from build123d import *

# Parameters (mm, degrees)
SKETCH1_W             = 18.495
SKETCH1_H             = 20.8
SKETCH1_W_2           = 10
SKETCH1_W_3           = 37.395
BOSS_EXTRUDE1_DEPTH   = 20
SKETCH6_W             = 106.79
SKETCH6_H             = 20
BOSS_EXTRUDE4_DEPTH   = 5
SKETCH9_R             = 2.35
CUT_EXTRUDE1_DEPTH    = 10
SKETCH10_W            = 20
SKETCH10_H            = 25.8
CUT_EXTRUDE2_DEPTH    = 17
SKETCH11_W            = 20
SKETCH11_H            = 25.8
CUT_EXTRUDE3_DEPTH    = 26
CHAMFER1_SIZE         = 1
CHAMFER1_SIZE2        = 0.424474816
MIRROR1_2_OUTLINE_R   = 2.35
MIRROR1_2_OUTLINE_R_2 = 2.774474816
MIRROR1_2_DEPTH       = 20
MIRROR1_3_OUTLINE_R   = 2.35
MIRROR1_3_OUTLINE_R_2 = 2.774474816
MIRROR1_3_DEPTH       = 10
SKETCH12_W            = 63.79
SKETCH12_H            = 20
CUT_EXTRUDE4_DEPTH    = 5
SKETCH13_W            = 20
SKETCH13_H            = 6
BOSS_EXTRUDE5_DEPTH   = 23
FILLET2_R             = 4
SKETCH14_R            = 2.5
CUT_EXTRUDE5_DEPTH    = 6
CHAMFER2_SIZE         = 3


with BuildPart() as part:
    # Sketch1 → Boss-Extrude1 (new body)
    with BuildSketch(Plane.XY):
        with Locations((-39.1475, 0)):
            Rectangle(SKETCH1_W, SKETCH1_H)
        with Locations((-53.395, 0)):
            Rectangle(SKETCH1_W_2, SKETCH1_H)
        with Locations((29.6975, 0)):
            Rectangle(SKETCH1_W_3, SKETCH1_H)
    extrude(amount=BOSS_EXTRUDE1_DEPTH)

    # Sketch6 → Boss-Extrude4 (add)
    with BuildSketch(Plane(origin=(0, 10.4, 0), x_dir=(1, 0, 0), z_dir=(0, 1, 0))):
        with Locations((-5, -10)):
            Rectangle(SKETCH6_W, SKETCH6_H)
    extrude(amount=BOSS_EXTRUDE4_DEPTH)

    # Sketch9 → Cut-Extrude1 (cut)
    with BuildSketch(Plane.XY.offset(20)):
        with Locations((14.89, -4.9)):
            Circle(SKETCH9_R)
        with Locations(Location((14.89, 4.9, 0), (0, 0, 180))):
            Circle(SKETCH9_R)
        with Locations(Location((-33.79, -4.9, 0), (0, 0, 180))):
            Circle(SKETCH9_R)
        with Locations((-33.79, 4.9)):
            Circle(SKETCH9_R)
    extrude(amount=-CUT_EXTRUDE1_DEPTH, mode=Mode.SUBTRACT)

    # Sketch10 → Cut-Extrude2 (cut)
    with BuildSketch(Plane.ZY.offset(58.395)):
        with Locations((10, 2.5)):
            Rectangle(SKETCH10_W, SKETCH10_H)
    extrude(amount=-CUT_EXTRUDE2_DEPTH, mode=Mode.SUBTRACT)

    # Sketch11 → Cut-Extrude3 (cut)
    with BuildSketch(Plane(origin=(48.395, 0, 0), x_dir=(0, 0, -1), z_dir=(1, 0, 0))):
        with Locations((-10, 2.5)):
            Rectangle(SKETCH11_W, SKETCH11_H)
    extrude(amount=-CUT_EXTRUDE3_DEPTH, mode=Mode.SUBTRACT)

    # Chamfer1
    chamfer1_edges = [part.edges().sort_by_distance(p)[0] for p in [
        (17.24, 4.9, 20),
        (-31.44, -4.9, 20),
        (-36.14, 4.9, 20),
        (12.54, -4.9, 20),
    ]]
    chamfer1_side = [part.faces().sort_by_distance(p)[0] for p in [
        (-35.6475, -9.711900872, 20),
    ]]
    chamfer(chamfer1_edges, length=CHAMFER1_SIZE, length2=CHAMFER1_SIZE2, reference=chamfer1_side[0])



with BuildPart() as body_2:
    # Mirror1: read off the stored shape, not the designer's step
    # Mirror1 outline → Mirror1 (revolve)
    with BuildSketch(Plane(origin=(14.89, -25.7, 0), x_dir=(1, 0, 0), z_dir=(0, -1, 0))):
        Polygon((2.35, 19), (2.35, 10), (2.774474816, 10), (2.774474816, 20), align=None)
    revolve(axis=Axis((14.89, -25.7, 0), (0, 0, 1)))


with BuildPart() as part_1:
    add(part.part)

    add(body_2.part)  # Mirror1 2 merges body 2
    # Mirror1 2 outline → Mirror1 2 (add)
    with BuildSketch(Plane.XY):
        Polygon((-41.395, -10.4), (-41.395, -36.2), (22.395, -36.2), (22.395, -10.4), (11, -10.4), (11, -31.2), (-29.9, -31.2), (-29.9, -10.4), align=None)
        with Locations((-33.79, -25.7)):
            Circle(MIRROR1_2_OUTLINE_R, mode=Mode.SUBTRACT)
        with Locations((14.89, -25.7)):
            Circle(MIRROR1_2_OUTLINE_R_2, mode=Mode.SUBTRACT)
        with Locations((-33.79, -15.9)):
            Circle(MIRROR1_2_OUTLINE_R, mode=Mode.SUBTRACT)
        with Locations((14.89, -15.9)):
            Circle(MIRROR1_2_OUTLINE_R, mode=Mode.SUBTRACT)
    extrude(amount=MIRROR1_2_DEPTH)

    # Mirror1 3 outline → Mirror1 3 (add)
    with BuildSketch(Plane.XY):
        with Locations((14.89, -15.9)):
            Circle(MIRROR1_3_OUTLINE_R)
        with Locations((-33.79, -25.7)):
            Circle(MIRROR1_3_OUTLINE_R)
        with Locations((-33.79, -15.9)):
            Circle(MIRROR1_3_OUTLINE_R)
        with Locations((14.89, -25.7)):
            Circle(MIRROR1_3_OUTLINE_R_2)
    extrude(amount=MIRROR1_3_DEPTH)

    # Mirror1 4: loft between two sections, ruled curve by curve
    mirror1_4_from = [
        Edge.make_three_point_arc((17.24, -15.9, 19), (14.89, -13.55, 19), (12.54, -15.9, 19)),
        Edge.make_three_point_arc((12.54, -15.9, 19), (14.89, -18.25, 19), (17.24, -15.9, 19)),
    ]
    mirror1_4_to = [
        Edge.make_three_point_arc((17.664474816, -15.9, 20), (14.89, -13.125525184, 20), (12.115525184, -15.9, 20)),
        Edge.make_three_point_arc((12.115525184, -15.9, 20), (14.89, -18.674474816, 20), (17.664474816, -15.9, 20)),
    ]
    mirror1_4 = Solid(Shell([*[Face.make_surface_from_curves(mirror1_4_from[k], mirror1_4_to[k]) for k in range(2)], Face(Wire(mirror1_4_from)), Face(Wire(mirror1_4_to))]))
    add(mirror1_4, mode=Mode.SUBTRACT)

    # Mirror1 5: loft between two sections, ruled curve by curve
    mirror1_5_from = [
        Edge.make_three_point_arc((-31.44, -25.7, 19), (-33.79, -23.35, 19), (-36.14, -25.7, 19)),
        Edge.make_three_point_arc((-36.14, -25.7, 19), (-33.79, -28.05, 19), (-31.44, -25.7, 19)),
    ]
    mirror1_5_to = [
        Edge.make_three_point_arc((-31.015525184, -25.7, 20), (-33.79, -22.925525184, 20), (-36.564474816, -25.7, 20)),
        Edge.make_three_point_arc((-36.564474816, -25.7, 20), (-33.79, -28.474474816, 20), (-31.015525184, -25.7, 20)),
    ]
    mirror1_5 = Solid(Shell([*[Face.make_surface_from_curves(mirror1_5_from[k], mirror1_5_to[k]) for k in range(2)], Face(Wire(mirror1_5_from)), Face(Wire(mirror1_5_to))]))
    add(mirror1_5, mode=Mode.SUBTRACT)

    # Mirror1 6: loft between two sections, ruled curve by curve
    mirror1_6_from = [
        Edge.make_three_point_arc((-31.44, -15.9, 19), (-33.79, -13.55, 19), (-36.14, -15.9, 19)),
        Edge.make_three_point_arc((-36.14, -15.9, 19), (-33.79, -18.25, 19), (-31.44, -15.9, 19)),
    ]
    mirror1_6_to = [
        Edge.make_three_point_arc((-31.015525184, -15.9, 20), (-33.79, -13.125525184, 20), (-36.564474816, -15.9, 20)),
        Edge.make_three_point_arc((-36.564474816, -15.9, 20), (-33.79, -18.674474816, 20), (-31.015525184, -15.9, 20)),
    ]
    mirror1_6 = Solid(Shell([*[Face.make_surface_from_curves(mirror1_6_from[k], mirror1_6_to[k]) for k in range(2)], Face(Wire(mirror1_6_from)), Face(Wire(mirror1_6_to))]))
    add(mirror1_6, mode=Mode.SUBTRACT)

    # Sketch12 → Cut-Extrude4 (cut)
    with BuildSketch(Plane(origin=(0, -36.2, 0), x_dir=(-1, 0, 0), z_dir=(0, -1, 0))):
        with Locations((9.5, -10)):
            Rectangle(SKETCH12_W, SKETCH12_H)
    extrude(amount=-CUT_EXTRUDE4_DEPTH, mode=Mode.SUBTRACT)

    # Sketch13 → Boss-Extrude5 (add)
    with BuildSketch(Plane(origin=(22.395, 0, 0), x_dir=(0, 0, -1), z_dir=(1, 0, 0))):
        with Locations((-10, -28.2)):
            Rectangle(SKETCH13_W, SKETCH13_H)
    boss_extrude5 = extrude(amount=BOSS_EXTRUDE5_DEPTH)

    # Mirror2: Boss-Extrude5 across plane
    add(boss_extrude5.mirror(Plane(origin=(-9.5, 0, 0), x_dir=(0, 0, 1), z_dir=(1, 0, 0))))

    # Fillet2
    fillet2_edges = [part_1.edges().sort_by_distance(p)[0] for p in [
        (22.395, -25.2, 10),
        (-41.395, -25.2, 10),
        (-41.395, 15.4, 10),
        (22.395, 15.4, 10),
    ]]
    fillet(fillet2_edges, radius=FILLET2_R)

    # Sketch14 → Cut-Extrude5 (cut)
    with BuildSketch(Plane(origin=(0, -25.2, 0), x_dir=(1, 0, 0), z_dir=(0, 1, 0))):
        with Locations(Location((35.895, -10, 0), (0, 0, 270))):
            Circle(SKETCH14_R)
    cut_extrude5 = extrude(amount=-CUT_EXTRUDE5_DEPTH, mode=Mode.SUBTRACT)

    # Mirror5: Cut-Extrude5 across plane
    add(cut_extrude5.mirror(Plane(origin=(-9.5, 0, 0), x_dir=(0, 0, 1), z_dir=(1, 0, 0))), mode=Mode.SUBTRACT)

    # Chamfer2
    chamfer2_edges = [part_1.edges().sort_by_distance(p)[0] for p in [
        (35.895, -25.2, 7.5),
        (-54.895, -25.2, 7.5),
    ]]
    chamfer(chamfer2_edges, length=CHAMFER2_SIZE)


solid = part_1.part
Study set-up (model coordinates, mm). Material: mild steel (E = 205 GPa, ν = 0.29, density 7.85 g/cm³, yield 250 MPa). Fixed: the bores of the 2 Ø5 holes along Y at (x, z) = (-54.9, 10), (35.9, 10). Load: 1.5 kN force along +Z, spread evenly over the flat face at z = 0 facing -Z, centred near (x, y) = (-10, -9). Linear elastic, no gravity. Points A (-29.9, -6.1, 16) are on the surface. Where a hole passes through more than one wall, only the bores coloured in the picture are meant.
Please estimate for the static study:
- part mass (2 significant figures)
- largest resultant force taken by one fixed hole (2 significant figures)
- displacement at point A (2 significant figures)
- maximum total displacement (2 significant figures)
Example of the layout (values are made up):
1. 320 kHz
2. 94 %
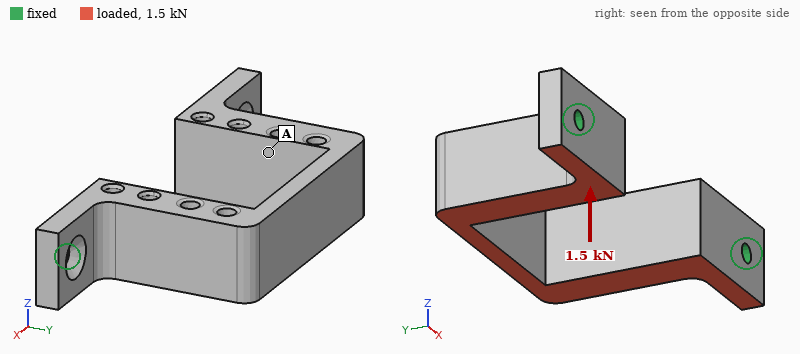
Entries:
1. 230 g
2. 750 N
3. 0.076 mm
4. 0.14 mm
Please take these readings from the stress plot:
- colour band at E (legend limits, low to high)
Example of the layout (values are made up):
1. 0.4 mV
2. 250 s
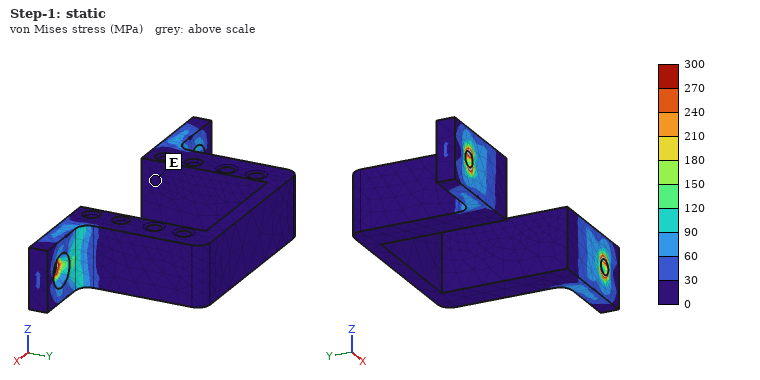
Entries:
1. 0 to 30 MPa
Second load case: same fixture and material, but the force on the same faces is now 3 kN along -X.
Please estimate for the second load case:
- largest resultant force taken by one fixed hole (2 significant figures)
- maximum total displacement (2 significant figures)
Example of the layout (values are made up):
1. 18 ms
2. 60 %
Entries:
1. 1.6 kN
2. 91 µm
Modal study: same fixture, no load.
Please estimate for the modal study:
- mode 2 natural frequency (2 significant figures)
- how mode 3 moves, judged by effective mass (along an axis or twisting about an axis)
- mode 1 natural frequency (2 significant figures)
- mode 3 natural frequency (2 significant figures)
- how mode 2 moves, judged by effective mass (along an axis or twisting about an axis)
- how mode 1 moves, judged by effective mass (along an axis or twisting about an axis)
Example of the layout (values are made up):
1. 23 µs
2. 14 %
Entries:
1. 2200 Hz
2. twisting about Y
3. 1200 Hz
4. 3400 Hz
5. along X
6. along Z
